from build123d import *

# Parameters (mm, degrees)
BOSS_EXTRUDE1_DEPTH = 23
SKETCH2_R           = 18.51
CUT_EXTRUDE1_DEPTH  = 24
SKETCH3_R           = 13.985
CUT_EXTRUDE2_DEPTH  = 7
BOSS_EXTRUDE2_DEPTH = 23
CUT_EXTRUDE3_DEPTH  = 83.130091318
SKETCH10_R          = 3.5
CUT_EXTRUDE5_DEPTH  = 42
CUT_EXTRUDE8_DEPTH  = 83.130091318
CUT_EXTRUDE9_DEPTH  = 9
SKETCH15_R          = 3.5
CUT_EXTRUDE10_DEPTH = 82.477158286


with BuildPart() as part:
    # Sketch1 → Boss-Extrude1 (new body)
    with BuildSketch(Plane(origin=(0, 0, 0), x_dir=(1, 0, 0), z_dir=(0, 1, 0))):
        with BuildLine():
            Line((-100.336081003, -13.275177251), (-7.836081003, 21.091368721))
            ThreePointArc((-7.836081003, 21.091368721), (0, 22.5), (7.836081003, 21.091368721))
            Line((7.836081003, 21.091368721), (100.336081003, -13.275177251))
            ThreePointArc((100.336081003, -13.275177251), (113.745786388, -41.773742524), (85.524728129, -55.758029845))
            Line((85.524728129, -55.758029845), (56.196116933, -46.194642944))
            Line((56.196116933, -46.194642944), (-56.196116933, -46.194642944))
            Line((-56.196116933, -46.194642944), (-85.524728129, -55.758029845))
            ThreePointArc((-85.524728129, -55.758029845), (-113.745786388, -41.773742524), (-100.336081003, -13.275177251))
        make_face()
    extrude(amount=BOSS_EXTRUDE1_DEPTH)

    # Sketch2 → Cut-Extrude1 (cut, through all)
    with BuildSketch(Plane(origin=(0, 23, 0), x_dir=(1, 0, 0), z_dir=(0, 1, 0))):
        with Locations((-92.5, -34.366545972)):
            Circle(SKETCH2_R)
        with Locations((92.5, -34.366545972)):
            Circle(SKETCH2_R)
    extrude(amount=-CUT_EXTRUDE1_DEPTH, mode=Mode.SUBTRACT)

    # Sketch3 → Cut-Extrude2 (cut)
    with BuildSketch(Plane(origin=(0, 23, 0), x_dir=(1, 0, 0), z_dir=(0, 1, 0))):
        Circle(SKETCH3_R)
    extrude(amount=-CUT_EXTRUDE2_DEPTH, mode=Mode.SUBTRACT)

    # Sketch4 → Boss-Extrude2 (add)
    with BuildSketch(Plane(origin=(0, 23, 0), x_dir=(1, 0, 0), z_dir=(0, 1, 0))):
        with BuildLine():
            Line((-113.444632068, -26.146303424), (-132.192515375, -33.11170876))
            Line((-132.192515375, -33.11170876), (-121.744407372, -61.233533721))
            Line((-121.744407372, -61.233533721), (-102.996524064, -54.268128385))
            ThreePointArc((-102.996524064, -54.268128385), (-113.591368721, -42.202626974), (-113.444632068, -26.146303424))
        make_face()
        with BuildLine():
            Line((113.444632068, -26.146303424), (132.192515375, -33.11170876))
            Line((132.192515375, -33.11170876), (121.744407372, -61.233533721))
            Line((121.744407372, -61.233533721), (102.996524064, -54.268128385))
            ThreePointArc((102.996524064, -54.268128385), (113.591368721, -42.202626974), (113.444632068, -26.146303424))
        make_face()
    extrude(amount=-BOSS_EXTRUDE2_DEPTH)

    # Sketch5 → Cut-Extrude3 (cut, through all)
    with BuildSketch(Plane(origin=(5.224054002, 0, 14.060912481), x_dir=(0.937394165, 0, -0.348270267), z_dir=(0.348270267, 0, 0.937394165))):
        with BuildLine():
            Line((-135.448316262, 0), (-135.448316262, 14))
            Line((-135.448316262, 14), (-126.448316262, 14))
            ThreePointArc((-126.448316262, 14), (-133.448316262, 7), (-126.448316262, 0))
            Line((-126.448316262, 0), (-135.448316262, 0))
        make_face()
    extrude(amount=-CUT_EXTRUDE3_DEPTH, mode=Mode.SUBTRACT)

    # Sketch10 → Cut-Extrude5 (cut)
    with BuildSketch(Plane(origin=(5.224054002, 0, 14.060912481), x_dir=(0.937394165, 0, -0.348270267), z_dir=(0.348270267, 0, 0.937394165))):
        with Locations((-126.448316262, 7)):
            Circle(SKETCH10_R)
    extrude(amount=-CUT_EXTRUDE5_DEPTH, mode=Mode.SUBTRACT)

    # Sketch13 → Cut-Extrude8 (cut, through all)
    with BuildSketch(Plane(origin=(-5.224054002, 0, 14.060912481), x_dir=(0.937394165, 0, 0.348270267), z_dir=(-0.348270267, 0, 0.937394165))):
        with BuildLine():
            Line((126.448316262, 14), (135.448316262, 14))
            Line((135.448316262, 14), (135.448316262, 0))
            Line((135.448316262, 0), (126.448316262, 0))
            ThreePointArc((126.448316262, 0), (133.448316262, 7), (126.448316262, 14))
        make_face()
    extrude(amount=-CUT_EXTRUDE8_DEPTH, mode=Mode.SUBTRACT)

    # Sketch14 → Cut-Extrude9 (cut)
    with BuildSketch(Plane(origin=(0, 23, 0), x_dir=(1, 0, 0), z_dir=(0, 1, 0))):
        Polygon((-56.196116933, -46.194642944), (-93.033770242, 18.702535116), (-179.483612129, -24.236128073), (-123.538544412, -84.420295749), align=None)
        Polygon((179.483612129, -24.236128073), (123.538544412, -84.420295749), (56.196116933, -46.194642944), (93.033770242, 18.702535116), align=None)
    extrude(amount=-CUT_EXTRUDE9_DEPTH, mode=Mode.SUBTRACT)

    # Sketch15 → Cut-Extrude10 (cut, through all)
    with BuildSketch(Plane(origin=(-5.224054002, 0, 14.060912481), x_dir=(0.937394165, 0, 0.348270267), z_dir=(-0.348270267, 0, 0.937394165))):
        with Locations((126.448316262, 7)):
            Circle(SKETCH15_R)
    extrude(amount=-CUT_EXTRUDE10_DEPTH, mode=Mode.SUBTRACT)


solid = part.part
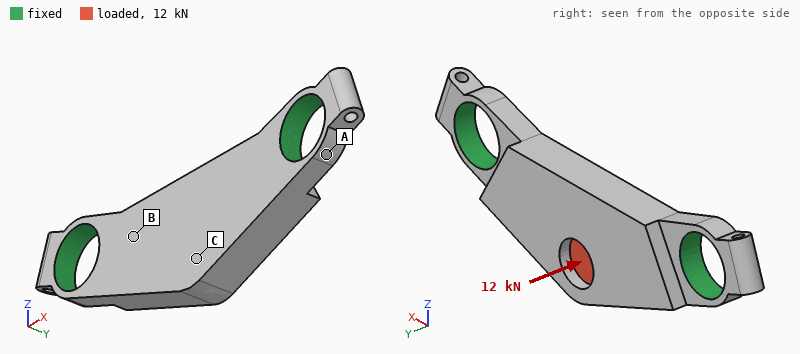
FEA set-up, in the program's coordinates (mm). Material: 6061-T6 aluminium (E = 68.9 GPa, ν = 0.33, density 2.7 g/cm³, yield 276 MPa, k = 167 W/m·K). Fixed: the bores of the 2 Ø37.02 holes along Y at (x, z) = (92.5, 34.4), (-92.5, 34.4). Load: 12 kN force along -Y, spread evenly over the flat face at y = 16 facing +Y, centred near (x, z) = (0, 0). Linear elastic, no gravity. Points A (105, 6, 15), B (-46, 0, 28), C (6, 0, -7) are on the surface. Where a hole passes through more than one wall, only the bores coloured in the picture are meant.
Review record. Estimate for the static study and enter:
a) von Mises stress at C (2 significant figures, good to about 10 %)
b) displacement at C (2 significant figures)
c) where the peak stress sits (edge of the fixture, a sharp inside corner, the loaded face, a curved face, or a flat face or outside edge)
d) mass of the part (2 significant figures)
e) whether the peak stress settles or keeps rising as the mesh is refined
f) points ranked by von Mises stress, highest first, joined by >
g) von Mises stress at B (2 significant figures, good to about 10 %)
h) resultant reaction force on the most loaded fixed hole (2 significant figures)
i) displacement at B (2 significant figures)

60 MPa
0.26 mm
edge of the fixture
570 g
keeps rising
C > B > A
34 MPa
8.9 kN
0.066 mm
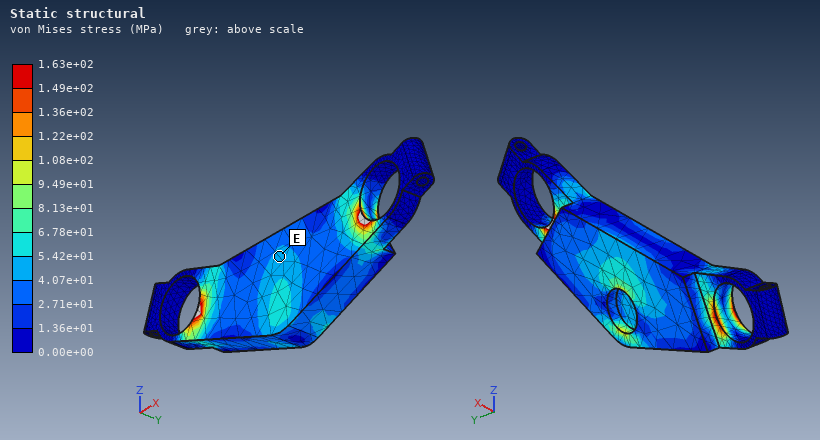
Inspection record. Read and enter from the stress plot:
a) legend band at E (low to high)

4.07e+01 to 5.42e+01 MPa
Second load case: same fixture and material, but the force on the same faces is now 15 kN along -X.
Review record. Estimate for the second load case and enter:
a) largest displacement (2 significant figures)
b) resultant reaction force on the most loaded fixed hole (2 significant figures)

19 µm
8.0 kN
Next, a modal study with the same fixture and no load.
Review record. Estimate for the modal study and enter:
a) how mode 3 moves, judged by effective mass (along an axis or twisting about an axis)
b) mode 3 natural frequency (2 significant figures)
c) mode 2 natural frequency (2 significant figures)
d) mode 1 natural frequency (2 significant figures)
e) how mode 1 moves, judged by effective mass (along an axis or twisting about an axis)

along Z
5900 Hz
4900 Hz
2600 Hz
along Y
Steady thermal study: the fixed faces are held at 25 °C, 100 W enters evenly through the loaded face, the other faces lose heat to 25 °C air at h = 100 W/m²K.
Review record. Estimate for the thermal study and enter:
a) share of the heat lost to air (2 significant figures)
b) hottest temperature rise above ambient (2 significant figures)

27 %
26 K
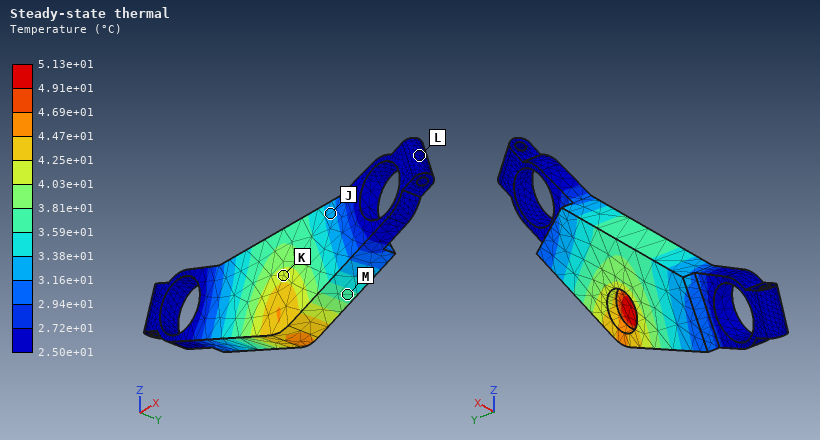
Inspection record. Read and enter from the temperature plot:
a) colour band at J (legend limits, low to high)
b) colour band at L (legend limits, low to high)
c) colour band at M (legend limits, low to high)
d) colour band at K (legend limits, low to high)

3.16e+01 to 3.38e+01 °C
2.50e+01 to 2.72e+01 °C
3.59e+01 to 3.81e+01 °C
4.03e+01 to 4.25e+01 °C
